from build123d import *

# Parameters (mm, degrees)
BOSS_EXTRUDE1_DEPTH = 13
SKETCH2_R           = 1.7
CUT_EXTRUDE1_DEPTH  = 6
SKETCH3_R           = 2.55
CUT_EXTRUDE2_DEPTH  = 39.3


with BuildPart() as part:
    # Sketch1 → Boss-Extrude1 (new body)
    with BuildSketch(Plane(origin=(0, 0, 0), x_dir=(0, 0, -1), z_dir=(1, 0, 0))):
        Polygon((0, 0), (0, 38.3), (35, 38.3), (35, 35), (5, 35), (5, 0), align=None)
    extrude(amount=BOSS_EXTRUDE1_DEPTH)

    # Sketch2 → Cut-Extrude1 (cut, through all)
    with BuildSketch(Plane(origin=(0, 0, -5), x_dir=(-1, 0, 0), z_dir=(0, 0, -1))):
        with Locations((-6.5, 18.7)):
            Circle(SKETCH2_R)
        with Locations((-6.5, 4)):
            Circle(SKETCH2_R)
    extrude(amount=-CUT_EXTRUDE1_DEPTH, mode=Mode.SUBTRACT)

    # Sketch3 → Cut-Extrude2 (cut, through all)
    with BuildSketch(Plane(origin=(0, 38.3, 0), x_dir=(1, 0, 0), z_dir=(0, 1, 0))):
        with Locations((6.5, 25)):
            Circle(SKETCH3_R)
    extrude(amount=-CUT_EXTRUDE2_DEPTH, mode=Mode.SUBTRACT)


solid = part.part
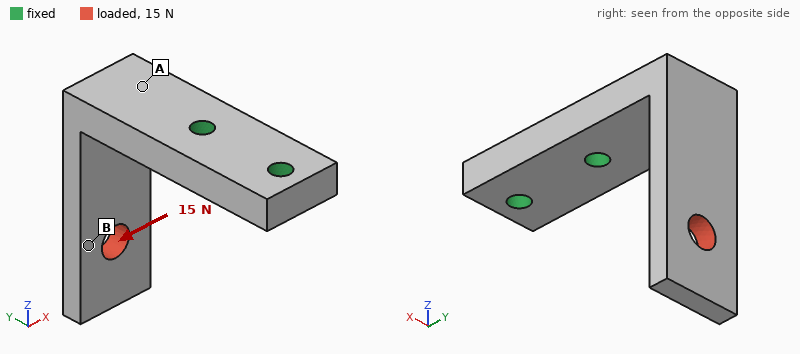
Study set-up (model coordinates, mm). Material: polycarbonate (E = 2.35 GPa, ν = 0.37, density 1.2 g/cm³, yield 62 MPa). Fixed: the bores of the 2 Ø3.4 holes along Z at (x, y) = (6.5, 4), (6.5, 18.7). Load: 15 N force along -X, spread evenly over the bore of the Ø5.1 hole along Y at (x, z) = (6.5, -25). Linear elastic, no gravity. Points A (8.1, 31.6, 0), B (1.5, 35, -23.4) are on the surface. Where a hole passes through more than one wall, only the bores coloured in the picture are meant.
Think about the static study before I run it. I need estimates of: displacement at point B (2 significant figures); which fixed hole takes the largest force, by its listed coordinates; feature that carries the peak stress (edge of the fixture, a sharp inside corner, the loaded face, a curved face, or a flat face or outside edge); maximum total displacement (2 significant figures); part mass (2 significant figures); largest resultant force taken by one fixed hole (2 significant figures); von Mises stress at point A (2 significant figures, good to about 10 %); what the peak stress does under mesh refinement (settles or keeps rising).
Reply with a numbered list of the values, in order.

1. 0.40 mm
2. (6.5, 18.7)
3. edge of the fixture
4. 0.61 mm
5. 4.3 g
6. 26 N
7. 5.3 MPa
8. keeps rising
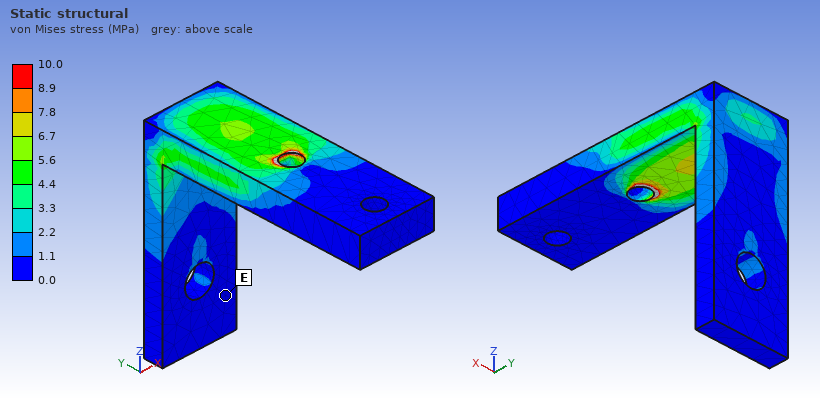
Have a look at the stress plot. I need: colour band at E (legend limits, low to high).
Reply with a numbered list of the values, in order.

1. 0.0 to 1.1 MPa
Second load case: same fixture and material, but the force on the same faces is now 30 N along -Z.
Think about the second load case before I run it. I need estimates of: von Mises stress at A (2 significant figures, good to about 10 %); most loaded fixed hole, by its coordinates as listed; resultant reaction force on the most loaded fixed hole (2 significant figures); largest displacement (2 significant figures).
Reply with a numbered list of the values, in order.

1. 2.7 MPa
2. (6.5, 18.7)
3. 37 N
4. 0.53 mm
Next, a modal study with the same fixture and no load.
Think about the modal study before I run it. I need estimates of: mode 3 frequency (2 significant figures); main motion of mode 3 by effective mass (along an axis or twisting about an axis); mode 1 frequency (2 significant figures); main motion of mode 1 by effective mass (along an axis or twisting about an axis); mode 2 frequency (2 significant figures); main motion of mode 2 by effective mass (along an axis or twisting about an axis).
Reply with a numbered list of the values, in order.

1. 1700 Hz
2. along Z
3. 590 Hz
4. along Y
5. 890 Hz
6. along X
